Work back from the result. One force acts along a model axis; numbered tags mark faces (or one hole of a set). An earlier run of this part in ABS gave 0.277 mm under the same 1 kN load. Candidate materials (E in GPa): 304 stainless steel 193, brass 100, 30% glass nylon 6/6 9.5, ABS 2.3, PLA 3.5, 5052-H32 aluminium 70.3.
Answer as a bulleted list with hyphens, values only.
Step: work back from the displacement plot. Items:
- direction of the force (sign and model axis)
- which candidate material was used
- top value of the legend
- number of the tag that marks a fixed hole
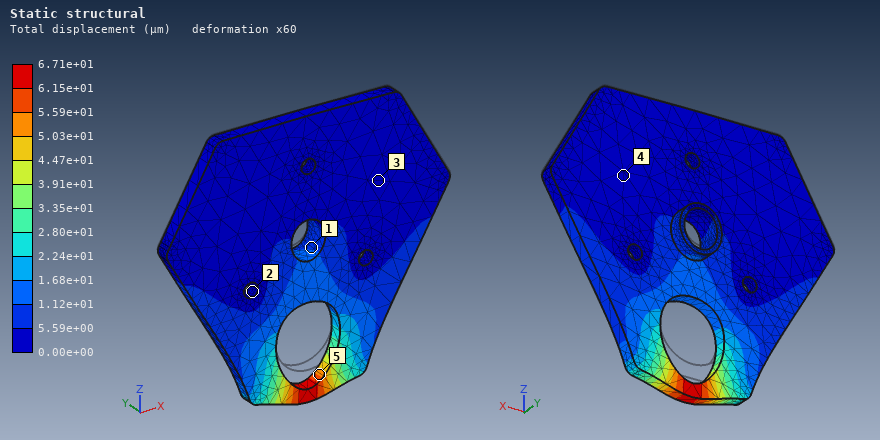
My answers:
- -Z
- 30% glass nylon 6/6
- 6.71e+01 µm
- 2
